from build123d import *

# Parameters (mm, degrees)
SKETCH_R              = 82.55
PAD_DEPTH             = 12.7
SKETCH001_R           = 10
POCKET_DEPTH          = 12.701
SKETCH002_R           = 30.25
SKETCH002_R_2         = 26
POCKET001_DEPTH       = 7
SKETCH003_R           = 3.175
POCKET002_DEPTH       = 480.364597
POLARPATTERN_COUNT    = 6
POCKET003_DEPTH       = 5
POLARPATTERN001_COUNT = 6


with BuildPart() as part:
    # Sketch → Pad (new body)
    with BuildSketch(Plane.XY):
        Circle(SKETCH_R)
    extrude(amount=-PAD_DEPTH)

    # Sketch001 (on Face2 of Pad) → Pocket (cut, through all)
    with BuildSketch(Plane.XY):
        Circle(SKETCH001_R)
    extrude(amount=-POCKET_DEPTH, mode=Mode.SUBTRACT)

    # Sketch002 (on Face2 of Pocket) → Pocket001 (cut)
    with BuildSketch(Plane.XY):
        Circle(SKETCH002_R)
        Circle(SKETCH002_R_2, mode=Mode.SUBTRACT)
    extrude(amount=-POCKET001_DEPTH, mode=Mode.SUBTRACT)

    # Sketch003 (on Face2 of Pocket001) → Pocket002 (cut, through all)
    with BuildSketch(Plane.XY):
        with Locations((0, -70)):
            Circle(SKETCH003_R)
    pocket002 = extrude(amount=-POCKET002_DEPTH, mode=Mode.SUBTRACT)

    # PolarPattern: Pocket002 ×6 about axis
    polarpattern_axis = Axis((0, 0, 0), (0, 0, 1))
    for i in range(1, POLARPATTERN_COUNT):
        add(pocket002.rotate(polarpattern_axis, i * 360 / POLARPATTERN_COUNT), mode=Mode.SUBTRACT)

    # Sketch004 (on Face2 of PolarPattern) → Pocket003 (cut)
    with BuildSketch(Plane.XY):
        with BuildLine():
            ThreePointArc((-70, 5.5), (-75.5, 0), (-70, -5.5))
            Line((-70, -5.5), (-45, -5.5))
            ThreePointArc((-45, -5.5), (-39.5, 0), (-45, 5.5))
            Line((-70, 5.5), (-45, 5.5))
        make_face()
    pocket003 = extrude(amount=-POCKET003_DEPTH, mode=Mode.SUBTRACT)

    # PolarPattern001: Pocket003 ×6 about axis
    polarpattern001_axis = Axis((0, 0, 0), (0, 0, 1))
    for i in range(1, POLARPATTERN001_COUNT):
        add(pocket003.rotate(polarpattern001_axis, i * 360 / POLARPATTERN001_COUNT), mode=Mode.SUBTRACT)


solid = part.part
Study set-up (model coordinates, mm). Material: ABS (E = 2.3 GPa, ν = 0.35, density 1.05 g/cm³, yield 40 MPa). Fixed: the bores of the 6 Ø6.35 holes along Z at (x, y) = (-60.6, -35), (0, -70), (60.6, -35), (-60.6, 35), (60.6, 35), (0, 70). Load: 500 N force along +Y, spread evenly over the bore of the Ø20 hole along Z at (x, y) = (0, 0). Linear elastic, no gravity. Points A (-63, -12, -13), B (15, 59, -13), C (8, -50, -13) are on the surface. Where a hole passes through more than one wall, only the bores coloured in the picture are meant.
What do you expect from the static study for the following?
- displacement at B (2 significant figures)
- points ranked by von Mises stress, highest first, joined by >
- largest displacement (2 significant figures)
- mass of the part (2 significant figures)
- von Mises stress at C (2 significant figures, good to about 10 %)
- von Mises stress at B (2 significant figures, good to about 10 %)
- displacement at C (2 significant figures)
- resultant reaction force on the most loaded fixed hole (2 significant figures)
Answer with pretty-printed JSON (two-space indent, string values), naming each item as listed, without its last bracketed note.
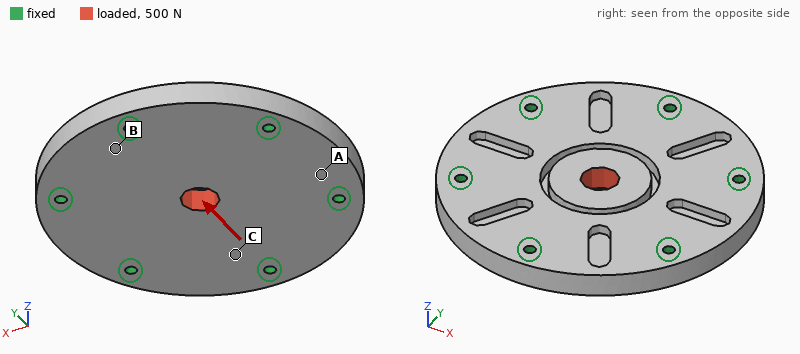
{
  "displacement at B": "4.6 µm",
  "points ranked by von Mises stress, highest first, joined by >": "C > B > A",
  "largest displacement": "22 µm",
  "mass of the part": "260 g",
  "von Mises stress at C": "0.46 MPa",
  "von Mises stress at B": "0.28 MPa",
  "displacement at C": "6.8 µm",
  "resultant reaction force on the most loaded fixed hole": "120 N"
}
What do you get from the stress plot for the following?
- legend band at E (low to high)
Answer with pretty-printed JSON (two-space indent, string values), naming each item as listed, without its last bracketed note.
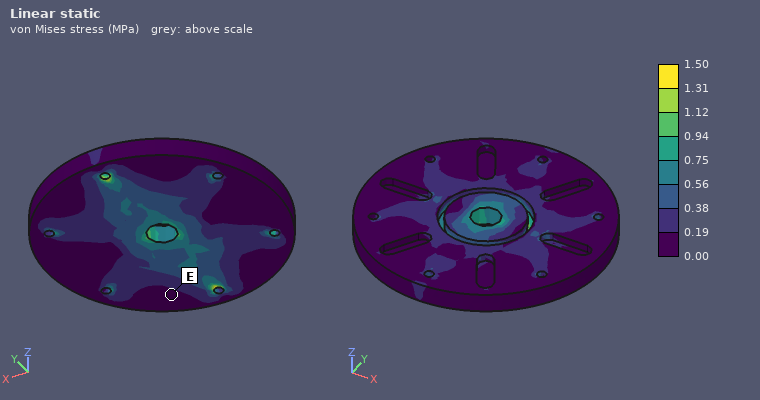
{
  "legend band at E": "0.00 to 0.19 MPa"
}
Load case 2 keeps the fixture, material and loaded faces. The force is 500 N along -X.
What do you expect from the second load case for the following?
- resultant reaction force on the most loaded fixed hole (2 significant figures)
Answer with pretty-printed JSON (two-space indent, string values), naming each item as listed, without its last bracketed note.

{
  "resultant reaction force on the most loaded fixed hole": "110 N"
}
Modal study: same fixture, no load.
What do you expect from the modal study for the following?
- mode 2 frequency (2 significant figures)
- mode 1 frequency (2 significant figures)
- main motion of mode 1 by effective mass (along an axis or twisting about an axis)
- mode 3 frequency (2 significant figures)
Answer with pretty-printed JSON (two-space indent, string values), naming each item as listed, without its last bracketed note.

{
  "mode 2 frequency": "2200 Hz",
  "mode 1 frequency": "1300 Hz",
  "main motion of mode 1 by effective mass": "along Z",
  "mode 3 frequency": "2200 Hz"
}
